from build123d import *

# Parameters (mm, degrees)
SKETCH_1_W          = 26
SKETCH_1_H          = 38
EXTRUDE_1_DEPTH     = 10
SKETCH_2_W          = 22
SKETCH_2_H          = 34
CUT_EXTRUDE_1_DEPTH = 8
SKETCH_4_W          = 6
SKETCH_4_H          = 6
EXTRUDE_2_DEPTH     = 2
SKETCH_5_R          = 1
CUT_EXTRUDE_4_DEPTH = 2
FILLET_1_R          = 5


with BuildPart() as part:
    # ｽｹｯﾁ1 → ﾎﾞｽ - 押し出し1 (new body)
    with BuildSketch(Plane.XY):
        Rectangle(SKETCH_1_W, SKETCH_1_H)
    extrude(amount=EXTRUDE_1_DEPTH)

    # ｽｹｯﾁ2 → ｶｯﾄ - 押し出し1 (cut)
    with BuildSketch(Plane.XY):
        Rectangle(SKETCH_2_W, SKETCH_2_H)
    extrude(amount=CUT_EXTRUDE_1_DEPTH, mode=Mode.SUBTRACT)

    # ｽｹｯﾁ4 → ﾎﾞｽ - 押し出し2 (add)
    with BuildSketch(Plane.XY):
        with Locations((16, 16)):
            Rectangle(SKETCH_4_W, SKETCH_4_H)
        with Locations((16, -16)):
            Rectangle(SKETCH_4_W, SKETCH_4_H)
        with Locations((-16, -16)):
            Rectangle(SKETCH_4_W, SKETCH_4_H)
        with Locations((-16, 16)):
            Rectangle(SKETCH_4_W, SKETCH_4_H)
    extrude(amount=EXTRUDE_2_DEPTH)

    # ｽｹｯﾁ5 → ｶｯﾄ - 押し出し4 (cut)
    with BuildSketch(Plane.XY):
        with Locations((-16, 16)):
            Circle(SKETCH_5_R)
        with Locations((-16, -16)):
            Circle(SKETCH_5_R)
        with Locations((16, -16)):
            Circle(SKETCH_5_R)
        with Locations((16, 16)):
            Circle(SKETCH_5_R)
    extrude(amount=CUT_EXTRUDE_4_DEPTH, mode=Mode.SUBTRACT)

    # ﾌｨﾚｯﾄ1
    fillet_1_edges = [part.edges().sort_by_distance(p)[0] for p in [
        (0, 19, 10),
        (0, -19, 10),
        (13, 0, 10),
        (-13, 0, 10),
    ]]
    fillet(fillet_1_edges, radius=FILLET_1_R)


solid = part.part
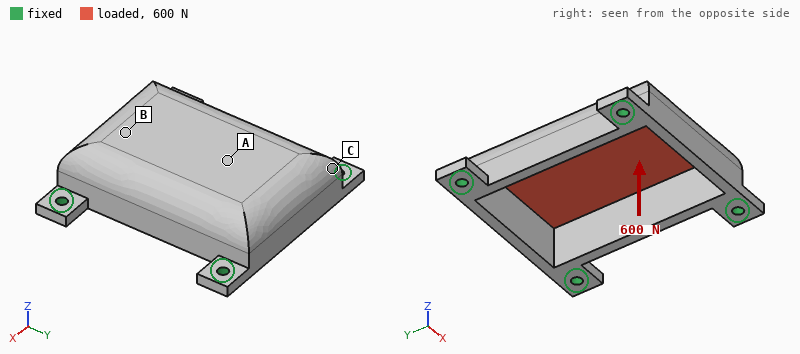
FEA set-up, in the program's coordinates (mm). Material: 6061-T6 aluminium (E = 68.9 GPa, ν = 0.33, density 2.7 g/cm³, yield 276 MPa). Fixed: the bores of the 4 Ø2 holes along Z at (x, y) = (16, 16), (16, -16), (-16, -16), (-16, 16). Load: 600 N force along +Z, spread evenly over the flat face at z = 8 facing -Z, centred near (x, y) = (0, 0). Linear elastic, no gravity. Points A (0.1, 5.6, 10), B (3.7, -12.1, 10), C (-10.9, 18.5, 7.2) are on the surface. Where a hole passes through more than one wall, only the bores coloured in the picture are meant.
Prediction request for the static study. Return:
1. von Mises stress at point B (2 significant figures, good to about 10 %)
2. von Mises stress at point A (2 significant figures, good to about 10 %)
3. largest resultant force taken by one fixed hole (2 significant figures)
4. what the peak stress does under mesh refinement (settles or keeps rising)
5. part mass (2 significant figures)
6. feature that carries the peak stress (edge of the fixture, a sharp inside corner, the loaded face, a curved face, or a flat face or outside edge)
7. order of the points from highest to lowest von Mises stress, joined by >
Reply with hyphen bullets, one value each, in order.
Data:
- 23 MPa
- 37 MPa
- 180 N
- keeps rising
- 9.5 g
- edge of the fixture
- A > B > C
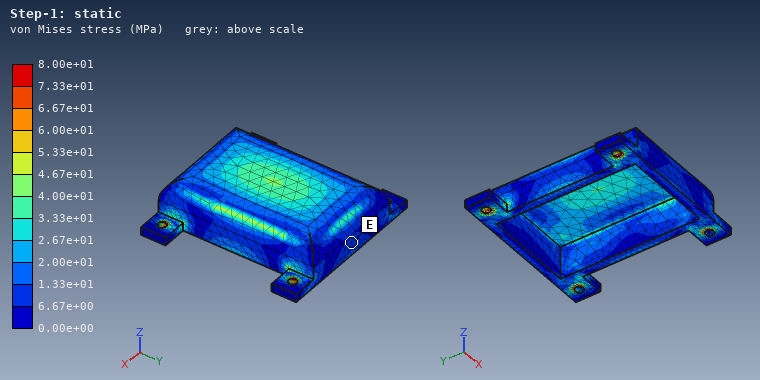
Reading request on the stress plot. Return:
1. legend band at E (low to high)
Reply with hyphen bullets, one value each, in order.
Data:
- 6.67e+00 to 1.33e+01 MPa
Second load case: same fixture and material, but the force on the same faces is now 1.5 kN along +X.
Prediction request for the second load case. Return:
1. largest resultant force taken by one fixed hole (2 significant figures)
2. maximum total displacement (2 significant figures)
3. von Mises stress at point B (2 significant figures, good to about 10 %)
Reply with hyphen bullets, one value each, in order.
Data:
- 420 N
- 25 µm
- 16 MPa
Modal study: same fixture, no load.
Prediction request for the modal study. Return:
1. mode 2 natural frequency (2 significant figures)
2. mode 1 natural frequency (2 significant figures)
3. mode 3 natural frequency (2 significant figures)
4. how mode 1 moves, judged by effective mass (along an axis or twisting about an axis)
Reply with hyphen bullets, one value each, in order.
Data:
- 15 kHz
- 12 kHz
- 16 kHz
- along Z
